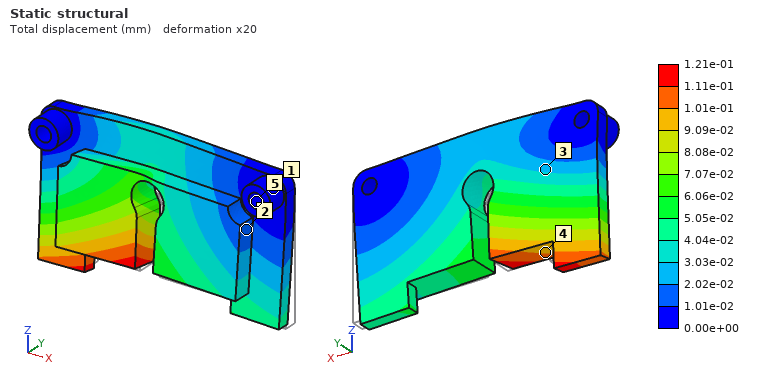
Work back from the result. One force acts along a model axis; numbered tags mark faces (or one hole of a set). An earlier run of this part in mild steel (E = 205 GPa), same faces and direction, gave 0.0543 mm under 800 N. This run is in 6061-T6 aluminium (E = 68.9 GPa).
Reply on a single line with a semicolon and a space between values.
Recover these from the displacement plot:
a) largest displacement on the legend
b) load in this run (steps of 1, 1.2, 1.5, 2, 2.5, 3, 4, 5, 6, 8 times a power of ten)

1.21e-01 mm; 600 N
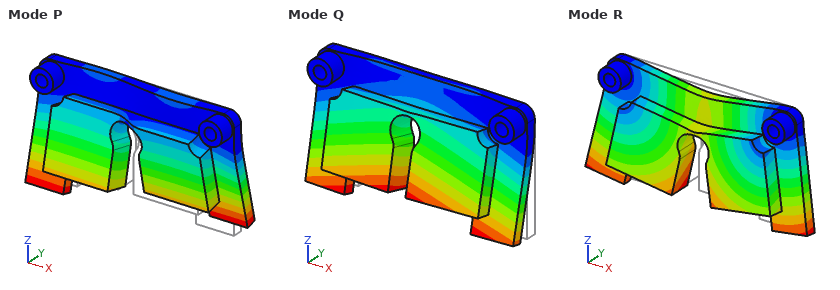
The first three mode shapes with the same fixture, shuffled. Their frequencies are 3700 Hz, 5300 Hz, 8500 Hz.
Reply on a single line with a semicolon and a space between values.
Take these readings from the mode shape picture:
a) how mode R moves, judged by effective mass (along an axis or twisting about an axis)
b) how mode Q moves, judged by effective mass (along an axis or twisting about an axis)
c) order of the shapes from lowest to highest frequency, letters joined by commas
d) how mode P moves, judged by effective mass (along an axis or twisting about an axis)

along Z; along Y; Q, P, R; twisting about Z
